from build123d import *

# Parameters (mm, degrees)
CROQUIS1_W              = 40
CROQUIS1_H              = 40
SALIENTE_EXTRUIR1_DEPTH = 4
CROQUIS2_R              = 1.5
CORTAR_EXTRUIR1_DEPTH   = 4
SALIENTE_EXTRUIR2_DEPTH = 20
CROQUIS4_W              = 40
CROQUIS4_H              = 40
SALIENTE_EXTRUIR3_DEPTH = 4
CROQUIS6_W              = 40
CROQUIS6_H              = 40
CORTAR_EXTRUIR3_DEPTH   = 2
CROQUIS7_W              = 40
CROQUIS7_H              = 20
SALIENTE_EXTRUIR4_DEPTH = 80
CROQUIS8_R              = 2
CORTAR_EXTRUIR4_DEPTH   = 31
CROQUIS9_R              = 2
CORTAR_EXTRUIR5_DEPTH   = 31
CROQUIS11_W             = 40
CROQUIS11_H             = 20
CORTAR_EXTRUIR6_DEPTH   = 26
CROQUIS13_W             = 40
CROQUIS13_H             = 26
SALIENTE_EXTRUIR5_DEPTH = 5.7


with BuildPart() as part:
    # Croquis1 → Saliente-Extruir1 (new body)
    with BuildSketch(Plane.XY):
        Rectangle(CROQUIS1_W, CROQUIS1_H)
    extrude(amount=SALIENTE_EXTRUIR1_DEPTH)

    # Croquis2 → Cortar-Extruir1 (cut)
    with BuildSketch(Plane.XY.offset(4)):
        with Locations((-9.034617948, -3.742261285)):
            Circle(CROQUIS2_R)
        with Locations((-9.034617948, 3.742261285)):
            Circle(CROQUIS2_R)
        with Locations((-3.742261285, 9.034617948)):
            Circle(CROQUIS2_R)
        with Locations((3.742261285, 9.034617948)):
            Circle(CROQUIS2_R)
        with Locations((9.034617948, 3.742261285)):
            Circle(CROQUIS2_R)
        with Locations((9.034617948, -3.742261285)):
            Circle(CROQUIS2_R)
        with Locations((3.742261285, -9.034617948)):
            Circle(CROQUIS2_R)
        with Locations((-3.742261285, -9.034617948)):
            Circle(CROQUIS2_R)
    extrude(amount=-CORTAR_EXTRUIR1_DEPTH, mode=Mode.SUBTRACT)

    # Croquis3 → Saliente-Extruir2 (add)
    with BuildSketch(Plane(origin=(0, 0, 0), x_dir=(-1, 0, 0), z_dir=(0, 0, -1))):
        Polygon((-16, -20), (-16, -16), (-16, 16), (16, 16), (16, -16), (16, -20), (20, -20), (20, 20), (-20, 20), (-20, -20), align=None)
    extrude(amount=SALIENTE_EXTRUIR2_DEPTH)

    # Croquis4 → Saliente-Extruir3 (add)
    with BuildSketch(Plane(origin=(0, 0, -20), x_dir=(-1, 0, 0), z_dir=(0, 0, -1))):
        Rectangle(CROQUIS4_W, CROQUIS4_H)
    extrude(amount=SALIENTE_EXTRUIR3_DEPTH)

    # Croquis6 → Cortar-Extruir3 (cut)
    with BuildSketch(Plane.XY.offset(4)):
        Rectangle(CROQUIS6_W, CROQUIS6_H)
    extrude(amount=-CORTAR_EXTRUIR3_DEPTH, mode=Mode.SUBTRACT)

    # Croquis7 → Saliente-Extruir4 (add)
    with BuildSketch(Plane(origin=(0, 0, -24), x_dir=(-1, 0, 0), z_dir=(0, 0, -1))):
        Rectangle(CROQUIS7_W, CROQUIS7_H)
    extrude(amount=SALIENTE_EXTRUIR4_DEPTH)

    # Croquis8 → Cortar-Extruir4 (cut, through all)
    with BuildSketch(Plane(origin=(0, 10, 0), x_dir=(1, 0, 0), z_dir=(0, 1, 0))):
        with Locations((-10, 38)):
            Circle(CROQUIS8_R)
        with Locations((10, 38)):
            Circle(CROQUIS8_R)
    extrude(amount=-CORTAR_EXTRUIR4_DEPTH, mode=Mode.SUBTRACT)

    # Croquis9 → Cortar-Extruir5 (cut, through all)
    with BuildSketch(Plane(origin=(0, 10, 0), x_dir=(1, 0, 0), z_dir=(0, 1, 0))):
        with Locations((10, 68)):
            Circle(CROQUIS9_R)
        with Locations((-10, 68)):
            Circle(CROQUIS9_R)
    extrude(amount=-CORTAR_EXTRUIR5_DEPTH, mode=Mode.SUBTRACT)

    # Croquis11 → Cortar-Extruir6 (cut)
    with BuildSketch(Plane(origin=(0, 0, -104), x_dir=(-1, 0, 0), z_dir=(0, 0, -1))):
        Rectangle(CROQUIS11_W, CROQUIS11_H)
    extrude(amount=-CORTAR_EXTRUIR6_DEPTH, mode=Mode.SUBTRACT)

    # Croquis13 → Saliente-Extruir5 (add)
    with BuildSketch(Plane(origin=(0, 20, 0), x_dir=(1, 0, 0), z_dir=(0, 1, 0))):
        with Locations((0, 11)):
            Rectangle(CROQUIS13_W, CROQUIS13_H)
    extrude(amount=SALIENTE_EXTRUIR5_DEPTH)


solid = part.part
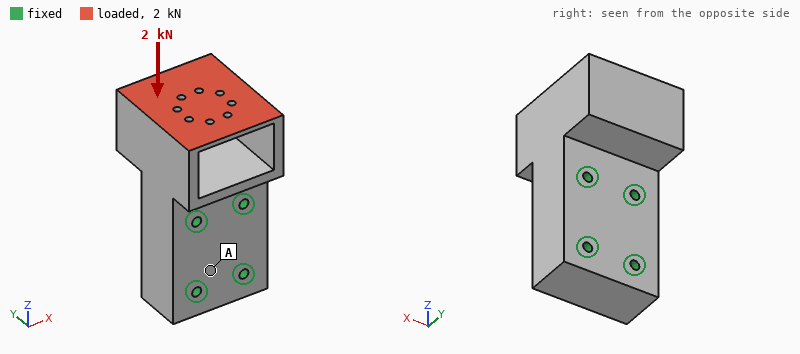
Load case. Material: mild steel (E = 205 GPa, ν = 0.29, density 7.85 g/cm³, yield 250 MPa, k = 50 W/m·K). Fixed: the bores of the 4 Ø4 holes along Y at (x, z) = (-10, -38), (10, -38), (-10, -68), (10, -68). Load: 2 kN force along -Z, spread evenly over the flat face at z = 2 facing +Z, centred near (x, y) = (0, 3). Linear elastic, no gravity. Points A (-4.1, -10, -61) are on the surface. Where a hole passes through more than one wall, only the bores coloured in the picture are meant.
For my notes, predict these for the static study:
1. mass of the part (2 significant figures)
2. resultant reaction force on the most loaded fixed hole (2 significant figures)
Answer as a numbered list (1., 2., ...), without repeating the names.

1. 520 g
2. 880 N
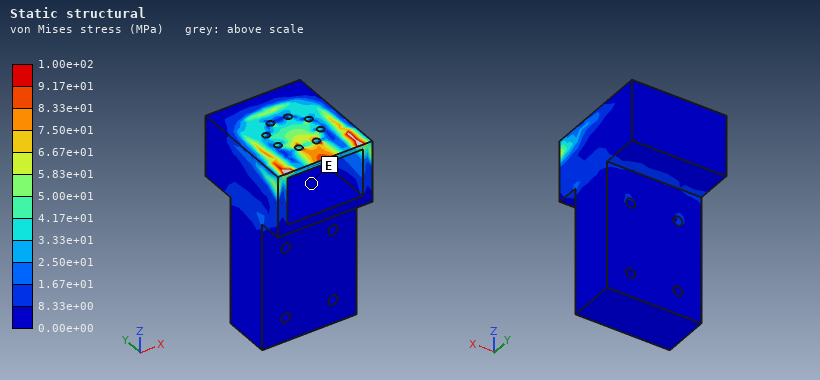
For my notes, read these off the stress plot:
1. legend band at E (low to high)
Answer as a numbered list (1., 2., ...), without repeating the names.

1. 0.00e+00 to 8.33e+00 MPa
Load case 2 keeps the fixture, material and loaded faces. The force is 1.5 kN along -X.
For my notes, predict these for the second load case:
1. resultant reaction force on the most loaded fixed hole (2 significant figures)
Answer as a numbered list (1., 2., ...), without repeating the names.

1. 2.1 kN
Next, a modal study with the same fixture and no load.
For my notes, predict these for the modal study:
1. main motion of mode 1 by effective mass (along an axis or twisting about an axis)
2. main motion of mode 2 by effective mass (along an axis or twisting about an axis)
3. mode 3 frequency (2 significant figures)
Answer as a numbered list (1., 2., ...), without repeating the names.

1. along Y
2. along X
3. 8800 Hz
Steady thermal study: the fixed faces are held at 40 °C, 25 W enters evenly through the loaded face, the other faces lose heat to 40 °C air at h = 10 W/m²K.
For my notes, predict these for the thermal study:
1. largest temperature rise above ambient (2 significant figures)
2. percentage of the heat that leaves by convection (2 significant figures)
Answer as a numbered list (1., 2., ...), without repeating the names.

1. 55 K
2. 9.7 %
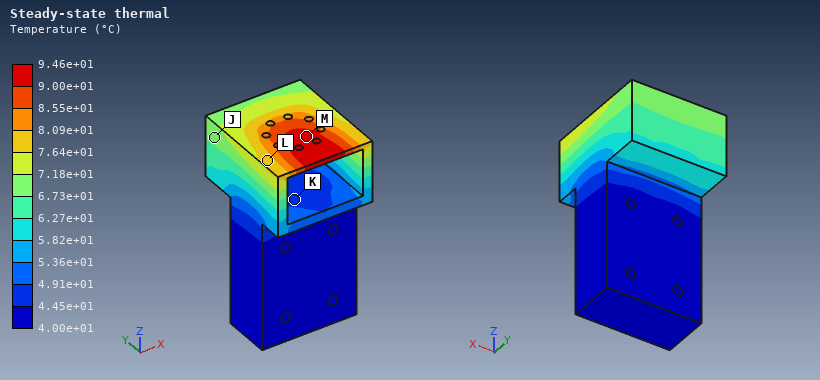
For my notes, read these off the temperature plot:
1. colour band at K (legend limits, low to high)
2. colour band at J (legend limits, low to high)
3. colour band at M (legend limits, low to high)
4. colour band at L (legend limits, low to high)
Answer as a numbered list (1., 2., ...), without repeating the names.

1. 4.45e+01 to 4.91e+01 °C
2. 6.73e+01 to 7.18e+01 °C
3. 9.00e+01 to 9.46e+01 °C
4. 7.64e+01 to 8.09e+01 °C
